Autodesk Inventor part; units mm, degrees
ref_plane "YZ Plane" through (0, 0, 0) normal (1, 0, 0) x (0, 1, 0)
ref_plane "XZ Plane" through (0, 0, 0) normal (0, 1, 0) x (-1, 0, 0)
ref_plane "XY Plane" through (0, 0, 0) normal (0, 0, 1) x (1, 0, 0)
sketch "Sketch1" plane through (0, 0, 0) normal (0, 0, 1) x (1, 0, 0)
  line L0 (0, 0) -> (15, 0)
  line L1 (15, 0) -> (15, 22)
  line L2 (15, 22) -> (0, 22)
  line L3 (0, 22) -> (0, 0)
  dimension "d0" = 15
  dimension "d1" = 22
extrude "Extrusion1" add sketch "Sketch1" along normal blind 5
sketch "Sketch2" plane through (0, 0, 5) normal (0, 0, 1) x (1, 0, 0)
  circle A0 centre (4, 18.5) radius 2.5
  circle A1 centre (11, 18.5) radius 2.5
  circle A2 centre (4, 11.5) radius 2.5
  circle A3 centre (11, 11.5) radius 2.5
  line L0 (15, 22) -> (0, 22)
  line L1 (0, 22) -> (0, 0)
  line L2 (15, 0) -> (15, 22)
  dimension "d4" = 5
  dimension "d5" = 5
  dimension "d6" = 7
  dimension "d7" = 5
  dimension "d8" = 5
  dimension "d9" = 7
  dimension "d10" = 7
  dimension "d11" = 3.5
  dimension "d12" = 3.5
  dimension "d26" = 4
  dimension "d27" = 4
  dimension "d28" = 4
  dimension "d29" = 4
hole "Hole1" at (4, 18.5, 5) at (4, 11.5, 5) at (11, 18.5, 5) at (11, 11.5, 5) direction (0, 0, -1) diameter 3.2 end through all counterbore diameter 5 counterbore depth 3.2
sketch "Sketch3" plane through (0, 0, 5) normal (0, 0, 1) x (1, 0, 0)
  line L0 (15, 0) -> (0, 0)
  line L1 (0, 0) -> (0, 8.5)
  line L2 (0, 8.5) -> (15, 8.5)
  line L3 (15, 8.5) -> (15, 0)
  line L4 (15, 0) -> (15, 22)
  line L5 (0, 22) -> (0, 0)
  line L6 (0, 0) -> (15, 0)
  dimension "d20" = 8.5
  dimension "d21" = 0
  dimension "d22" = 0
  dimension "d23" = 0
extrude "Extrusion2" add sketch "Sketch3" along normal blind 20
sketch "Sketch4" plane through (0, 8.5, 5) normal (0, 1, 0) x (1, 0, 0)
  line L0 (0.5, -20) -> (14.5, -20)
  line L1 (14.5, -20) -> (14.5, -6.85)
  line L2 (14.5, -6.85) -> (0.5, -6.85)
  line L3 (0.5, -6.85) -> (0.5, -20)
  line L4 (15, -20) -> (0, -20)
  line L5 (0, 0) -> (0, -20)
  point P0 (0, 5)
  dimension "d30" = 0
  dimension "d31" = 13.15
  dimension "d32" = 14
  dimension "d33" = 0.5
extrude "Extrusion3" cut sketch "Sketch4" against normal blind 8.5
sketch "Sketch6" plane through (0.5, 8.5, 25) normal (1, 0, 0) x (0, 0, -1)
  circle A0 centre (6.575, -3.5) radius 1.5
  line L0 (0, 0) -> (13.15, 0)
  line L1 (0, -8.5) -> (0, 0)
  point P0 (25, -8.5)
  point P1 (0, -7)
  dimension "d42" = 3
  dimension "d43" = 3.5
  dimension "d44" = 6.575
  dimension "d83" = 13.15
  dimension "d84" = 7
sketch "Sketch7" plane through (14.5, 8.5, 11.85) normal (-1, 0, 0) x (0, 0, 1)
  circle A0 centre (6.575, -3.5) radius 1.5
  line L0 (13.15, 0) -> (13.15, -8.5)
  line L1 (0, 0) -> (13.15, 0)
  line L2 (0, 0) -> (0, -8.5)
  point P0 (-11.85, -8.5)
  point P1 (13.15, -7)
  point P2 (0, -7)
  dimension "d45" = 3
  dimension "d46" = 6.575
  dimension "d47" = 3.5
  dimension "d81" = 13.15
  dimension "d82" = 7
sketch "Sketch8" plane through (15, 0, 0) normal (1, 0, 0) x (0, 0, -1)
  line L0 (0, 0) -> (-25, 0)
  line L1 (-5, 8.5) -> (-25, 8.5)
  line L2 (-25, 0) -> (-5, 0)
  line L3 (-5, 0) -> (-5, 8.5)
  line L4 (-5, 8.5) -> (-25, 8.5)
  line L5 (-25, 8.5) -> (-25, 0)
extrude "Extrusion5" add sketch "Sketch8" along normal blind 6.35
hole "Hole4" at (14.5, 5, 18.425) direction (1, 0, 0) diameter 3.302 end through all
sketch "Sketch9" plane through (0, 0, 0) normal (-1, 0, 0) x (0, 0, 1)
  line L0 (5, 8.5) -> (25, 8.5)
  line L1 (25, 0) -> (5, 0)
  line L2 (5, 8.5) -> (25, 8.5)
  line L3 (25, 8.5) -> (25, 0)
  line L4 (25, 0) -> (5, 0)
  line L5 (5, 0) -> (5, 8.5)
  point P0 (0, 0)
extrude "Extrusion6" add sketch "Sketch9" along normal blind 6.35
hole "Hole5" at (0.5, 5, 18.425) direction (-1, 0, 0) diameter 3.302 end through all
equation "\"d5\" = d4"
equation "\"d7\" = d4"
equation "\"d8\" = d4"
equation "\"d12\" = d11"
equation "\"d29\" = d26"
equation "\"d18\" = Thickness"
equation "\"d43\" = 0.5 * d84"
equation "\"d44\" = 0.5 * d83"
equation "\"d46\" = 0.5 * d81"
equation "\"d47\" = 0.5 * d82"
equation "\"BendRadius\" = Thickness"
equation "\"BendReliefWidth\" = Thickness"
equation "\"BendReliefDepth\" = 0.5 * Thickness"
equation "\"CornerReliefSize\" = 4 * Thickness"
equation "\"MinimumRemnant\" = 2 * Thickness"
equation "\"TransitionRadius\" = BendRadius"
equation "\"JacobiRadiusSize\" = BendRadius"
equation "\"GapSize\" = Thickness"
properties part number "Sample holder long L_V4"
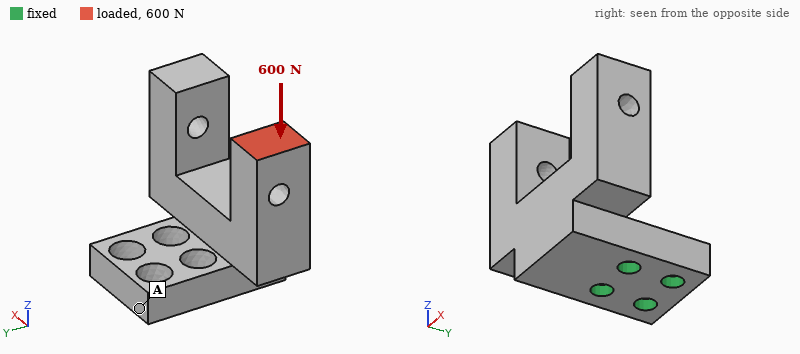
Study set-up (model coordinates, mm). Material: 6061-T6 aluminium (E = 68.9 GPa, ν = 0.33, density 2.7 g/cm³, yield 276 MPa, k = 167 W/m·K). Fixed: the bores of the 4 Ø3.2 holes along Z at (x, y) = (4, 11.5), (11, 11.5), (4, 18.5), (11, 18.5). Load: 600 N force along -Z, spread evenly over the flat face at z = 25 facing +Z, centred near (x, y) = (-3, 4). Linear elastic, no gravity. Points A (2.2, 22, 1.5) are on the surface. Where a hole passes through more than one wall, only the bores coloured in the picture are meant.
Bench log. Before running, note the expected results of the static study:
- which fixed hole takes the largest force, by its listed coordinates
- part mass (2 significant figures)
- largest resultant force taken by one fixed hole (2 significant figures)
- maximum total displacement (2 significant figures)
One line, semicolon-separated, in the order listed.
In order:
(4, 11.5); 12 g; 1.2 kN; 0.12 mm
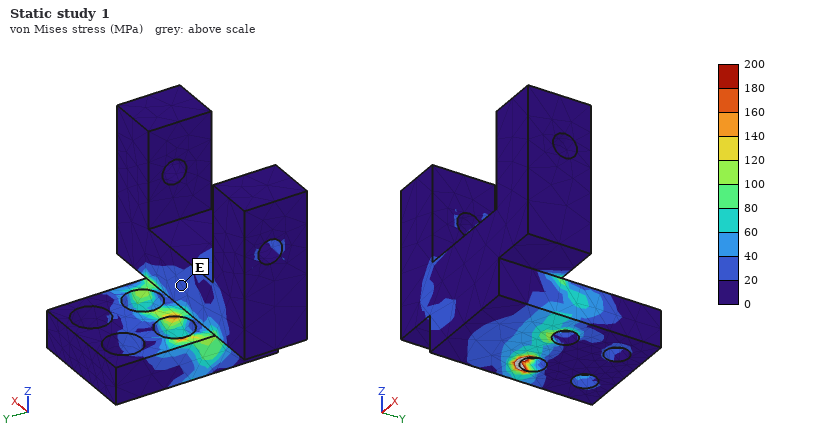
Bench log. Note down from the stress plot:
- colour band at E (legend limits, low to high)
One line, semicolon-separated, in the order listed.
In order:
20 to 40 MPa
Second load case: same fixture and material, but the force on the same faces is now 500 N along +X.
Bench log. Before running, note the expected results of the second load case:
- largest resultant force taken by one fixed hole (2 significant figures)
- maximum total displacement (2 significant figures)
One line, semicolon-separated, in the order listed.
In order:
1.4 kN; 0.21 mm
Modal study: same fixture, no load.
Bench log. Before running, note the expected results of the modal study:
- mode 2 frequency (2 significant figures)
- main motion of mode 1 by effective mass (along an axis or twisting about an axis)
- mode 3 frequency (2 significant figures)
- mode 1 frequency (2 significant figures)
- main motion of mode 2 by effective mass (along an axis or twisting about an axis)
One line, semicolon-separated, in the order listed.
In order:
5600 Hz; along Y; 9500 Hz; 4000 Hz; along X
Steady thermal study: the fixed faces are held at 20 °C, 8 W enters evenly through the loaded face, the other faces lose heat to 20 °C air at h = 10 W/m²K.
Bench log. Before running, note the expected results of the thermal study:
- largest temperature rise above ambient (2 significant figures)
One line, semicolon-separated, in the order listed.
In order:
25 K
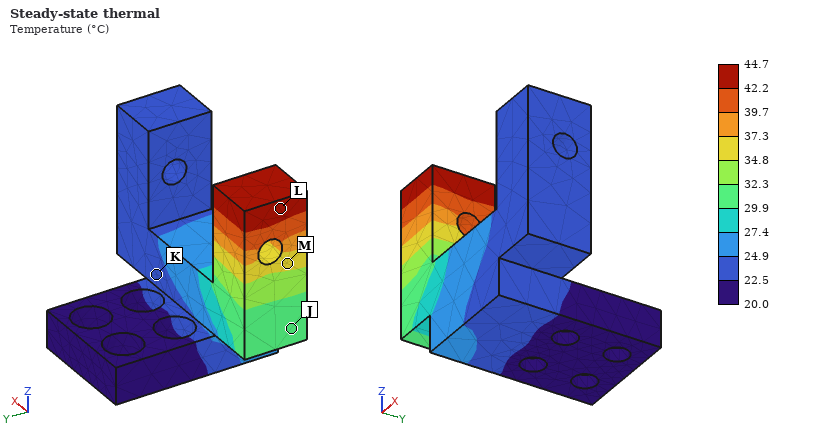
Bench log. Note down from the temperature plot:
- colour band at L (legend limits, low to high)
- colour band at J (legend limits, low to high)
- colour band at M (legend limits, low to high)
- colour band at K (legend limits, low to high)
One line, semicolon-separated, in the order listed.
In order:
42.2 to 44.7 °C; 29.9 to 32.3 °C; 34.8 to 37.3 °C; 22.5 to 24.9 °C
